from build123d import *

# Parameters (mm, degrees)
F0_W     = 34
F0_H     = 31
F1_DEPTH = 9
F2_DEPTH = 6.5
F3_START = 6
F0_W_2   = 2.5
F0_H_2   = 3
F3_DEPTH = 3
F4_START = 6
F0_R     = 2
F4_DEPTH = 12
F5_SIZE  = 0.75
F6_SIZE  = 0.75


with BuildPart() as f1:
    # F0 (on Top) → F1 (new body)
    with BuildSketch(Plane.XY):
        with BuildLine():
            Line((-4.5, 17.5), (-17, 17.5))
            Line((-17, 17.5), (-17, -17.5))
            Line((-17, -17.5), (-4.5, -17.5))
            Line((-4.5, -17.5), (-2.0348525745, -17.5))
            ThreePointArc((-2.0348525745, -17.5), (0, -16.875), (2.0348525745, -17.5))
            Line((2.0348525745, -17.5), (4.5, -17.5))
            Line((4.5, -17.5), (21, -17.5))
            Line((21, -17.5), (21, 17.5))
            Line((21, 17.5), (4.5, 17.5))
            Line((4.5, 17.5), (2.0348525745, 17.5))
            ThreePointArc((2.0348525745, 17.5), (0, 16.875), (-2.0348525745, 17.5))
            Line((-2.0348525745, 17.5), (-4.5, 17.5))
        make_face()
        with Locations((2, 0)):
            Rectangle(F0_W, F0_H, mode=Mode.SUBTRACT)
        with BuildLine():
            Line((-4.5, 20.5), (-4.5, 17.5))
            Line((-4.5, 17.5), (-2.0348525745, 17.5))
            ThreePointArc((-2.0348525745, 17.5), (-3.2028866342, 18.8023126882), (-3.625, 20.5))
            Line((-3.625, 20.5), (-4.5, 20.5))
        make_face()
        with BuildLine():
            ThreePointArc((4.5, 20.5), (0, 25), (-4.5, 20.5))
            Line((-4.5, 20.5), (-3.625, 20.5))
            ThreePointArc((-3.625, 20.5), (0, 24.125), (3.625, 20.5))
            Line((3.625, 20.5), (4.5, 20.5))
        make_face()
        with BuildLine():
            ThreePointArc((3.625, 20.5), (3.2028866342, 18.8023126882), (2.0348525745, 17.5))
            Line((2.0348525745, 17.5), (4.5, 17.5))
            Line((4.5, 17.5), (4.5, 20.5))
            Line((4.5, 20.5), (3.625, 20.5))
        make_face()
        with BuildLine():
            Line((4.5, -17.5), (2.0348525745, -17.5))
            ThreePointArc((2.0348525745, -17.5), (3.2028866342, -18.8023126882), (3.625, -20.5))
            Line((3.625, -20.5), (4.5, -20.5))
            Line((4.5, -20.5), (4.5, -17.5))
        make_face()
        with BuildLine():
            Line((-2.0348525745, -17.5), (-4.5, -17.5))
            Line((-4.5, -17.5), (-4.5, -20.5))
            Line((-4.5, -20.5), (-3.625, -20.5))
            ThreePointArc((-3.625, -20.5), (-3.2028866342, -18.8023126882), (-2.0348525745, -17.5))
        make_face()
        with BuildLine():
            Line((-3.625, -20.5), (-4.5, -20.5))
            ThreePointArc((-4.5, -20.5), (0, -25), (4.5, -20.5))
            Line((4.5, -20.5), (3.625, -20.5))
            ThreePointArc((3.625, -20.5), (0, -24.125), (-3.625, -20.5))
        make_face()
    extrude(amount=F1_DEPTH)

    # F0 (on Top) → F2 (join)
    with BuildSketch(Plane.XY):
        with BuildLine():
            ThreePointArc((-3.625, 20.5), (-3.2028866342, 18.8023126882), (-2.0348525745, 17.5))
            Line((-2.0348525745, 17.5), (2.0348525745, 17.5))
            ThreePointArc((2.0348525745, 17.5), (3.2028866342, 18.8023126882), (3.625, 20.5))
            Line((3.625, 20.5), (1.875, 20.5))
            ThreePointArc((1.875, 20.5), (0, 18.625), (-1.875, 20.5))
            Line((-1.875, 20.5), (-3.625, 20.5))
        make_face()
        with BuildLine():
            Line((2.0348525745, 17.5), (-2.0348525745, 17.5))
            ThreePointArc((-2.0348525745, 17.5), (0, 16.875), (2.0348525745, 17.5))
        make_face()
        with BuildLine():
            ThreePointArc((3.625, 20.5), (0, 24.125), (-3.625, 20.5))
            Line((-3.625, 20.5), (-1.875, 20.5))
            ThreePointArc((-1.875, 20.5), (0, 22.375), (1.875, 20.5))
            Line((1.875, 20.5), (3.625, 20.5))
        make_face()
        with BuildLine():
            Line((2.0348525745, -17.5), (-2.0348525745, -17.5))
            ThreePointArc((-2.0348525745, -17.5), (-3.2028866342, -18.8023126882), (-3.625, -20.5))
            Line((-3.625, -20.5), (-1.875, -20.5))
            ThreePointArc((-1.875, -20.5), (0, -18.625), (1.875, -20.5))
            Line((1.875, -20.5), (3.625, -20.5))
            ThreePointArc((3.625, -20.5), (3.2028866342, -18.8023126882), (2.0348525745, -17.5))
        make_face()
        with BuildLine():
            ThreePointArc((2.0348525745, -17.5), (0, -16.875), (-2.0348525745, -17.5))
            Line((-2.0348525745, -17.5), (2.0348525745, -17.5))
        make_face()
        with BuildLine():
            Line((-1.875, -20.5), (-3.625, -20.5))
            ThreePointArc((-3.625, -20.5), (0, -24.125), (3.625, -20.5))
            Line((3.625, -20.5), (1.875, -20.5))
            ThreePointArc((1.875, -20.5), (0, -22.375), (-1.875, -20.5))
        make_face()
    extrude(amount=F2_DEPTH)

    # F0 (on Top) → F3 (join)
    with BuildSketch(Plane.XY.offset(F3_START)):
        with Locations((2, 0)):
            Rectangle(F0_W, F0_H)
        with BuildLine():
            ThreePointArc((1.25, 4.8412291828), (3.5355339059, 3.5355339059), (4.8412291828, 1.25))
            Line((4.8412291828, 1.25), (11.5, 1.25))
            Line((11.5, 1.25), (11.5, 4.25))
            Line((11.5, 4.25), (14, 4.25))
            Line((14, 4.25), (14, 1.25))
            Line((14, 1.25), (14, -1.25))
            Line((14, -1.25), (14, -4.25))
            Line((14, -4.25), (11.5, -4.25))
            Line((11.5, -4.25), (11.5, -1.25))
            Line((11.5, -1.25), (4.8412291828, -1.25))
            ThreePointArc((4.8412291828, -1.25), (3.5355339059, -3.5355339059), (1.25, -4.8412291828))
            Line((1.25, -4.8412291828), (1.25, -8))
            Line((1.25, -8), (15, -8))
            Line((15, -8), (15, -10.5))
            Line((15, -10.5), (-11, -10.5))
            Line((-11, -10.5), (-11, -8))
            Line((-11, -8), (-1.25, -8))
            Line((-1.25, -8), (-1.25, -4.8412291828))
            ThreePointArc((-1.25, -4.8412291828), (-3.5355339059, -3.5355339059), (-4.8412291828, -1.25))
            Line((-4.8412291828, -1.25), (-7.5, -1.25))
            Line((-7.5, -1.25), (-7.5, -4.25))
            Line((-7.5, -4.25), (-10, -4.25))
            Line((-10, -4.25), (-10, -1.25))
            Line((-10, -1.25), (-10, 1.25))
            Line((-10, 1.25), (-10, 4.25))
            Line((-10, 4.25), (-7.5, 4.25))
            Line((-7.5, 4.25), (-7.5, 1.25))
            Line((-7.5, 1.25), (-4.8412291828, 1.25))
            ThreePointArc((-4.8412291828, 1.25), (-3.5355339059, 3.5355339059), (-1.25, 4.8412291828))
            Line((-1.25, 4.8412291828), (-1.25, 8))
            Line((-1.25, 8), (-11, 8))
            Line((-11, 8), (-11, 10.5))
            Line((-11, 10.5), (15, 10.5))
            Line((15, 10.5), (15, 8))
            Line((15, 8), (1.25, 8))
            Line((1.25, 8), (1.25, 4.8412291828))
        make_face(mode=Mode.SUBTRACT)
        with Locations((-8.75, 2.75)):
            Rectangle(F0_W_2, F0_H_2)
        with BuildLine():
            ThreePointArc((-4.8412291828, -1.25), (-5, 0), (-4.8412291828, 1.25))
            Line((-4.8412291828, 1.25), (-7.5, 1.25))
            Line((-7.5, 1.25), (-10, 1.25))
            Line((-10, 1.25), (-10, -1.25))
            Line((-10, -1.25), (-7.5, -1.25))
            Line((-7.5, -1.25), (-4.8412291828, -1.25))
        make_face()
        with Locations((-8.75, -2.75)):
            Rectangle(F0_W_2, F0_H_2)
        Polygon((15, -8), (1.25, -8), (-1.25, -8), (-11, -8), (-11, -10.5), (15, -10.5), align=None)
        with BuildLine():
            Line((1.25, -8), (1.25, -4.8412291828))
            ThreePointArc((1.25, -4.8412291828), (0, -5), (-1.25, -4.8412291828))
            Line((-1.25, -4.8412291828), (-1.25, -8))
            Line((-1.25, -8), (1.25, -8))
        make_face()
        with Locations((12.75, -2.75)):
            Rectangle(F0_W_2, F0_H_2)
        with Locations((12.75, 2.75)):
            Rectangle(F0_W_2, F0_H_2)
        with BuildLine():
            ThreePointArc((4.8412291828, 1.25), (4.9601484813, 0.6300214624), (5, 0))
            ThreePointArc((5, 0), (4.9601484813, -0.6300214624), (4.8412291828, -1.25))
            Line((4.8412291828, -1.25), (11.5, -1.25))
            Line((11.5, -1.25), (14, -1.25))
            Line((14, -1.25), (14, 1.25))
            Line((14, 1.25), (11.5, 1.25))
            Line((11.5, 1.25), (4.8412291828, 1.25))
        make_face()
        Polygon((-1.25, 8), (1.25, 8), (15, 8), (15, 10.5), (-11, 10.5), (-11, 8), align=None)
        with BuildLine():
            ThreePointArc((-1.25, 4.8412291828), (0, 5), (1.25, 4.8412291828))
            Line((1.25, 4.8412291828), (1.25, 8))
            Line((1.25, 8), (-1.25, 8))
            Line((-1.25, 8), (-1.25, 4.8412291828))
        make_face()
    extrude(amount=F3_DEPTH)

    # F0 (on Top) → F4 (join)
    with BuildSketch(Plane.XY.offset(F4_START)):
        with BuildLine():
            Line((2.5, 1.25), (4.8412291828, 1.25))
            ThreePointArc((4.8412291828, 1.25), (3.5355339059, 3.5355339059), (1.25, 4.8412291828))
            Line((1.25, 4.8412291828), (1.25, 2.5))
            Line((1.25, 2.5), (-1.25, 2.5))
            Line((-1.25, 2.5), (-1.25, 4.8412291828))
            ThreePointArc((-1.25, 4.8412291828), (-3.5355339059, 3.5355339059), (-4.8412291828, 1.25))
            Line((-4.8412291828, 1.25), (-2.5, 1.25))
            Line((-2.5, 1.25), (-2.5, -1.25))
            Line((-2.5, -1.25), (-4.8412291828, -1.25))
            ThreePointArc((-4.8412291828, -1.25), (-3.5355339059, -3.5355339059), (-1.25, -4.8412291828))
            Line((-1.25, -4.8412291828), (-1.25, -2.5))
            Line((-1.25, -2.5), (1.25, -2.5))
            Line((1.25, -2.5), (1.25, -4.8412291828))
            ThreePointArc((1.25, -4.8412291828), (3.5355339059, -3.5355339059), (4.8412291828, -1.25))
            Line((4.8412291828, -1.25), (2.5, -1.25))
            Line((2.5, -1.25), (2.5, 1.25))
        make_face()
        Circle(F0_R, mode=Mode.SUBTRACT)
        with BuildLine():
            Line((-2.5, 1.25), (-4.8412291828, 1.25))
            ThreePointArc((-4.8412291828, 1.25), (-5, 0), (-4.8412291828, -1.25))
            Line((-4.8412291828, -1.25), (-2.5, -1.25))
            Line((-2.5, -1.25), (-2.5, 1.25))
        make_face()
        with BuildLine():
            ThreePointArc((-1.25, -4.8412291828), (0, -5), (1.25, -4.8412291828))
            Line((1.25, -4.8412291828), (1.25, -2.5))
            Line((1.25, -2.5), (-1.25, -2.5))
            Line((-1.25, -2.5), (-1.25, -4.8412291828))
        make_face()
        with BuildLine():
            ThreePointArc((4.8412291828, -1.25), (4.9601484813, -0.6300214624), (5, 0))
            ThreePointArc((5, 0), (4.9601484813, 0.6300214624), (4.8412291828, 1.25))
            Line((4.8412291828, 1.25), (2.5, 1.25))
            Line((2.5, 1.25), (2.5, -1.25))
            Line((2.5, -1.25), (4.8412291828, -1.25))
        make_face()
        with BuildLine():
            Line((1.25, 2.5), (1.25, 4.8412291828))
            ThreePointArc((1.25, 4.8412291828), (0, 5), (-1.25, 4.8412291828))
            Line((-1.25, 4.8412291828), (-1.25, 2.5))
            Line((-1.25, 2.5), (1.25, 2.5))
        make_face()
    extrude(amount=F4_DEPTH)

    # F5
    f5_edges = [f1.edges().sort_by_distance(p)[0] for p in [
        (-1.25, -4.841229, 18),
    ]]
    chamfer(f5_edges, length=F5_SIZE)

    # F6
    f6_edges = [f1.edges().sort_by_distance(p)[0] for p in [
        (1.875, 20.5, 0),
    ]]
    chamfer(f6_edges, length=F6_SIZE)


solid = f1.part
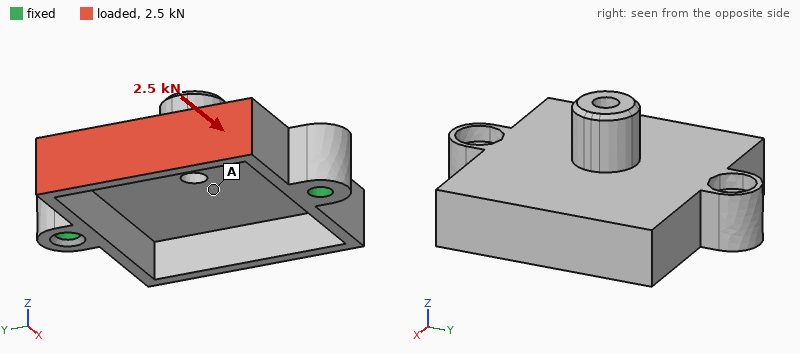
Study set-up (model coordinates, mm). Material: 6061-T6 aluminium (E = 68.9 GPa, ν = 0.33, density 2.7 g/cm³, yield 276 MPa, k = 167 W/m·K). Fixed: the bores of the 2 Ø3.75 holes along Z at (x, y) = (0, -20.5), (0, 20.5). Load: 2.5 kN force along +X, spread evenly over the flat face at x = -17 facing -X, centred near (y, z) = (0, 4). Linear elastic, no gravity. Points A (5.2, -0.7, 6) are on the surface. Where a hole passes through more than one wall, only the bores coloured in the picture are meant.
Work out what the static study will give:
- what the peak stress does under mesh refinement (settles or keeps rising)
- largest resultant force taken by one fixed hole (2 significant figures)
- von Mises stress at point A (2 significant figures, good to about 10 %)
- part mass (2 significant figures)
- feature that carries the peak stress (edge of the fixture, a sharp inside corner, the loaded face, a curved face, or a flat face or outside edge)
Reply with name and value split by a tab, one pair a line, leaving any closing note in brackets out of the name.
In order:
what the peak stress does under mesh refinement	keeps rising
largest resultant force taken by one fixed hole	1.3 kN
von Mises stress at point A	12 MPa
part mass	19 g
feature that carries the peak stress	edge of the fixture
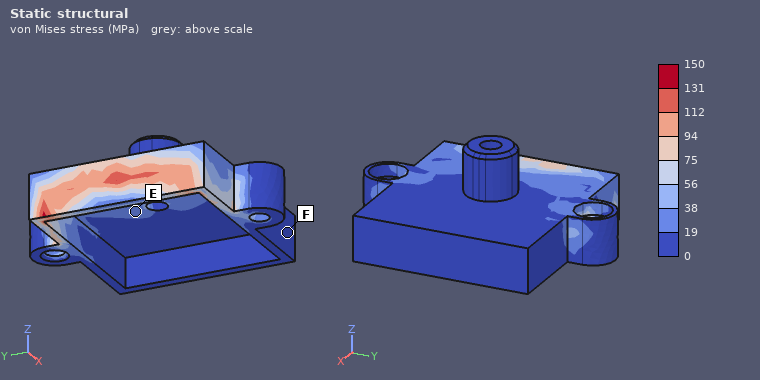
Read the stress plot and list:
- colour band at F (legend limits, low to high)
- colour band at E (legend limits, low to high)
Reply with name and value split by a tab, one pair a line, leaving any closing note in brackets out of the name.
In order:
colour band at F	0 to 19 MPa
colour band at E	19 to 38 MPa
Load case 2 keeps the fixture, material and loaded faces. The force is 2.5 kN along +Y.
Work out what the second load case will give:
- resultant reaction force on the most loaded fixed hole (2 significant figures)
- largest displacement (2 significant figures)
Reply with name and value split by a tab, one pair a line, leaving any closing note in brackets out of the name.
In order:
resultant reaction force on the most loaded fixed hole	1.7 kN
largest displacement	90 µm
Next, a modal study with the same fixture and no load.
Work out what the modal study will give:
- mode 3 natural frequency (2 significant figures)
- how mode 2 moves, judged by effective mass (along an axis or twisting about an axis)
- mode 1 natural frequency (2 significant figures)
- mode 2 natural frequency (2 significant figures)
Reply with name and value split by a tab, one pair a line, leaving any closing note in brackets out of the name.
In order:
mode 3 natural frequency	11 kHz
how mode 2 moves, judged by effective mass	along Z
mode 1 natural frequency	6200 Hz
mode 2 natural frequency	9300 Hz
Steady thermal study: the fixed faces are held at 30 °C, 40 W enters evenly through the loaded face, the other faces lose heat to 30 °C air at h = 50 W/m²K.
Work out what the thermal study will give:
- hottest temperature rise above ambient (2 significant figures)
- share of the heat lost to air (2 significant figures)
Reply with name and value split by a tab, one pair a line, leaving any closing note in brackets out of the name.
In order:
hottest temperature rise above ambient	48 K
share of the heat lost to air	10 %
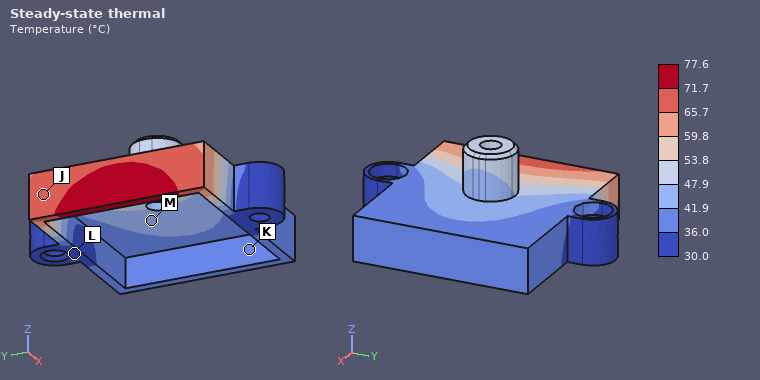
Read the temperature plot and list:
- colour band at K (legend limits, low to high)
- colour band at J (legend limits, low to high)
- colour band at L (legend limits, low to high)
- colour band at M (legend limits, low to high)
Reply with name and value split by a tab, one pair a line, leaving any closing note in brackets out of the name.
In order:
colour band at K	36.0 to 41.9 °C
colour band at J	65.7 to 71.7 °C
colour band at L	30.0 to 36.0 °C
colour band at M	41.9 to 47.9 °C
